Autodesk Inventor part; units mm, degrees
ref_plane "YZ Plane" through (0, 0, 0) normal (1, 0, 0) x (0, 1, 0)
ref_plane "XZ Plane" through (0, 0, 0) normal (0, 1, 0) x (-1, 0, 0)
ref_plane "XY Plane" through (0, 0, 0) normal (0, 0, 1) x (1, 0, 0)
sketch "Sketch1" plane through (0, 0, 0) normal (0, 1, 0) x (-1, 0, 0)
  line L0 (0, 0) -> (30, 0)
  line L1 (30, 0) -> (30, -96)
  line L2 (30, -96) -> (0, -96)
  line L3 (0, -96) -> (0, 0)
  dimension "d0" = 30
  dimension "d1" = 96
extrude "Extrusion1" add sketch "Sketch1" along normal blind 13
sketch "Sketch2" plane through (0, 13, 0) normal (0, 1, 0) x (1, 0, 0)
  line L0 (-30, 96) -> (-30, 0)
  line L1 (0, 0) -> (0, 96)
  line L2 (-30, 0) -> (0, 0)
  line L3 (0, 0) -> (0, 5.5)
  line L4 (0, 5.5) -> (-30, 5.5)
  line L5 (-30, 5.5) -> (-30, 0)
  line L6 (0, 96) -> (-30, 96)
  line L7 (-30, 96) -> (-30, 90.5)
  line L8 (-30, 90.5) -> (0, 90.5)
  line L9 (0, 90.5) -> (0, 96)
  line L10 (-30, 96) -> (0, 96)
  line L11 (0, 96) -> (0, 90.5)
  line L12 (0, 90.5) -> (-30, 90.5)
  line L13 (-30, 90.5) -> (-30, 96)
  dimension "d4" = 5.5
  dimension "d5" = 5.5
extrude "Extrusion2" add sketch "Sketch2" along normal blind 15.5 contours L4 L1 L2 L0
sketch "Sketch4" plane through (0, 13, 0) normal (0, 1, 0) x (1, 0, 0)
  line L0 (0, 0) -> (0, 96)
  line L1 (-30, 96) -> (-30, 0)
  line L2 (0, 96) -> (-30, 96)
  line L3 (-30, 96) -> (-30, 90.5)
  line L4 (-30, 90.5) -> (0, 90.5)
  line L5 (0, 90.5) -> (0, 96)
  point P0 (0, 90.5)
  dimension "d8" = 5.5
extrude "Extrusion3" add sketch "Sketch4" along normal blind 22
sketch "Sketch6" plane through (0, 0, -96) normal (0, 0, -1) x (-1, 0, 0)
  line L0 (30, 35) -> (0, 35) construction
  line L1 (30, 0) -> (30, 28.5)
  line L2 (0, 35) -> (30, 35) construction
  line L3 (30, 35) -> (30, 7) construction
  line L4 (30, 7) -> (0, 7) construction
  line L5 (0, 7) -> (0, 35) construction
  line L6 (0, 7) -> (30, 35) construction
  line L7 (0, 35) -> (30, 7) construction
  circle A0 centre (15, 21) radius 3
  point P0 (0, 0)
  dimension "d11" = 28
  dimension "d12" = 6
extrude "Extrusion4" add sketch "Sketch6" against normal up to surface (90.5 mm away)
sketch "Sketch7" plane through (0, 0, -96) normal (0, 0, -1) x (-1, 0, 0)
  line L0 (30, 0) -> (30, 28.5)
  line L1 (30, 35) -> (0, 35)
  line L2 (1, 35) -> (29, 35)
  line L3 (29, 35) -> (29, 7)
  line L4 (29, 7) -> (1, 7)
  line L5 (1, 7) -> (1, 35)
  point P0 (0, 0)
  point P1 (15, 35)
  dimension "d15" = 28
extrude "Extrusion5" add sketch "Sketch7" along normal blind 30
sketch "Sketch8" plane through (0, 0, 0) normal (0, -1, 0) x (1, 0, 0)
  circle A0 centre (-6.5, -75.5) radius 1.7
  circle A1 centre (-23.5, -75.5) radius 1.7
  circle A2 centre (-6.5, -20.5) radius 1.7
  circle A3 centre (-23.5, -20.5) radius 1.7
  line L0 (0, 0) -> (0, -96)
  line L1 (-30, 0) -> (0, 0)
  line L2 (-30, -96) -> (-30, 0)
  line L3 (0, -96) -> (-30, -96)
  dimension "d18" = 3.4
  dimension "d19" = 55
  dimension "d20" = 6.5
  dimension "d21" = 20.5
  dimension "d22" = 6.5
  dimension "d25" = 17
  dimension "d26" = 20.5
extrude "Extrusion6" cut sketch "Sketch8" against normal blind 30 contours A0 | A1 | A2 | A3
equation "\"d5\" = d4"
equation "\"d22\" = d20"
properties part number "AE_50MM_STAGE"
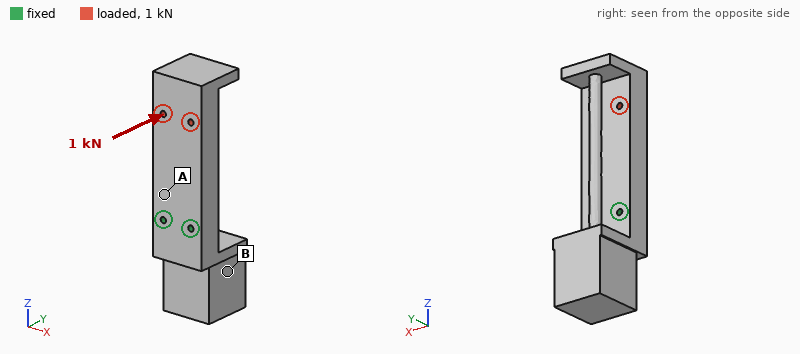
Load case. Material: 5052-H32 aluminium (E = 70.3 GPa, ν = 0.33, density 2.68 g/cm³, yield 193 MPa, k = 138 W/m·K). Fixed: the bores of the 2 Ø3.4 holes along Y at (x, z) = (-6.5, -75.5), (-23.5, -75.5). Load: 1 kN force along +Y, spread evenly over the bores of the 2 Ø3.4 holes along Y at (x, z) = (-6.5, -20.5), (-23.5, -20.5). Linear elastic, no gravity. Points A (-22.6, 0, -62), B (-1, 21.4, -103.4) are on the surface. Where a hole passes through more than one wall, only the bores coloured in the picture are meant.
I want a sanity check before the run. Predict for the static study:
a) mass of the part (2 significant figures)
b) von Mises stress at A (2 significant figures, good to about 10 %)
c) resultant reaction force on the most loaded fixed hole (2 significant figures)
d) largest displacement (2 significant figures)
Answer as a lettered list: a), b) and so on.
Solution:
a) 190 g
b) 42 MPa
c) 510 N
d) 0.20 mm
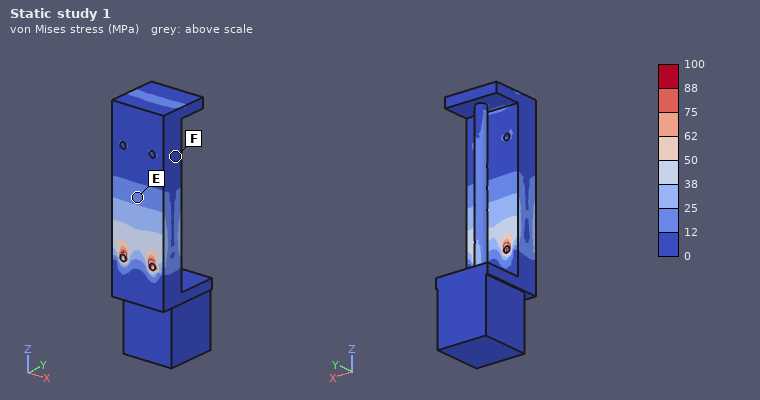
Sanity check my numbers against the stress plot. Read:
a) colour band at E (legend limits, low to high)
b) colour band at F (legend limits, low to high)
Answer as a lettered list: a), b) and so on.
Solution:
a) 12 to 25 MPa
b) 0 to 12 MPa
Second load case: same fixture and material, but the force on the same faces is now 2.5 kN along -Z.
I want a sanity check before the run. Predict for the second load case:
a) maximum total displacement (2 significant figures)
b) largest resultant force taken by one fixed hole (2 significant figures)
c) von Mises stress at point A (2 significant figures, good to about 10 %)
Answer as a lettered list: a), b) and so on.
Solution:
a) 7.4 µm
b) 1.3 kN
c) 7.2 MPa
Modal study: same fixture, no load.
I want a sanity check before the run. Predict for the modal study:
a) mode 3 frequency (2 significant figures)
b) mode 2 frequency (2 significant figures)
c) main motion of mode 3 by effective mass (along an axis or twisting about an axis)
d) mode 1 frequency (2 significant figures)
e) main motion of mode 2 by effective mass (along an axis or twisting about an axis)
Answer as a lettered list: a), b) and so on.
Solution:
a) 3000 Hz
b) 2500 Hz
c) along X
d) 1600 Hz
e) along Y
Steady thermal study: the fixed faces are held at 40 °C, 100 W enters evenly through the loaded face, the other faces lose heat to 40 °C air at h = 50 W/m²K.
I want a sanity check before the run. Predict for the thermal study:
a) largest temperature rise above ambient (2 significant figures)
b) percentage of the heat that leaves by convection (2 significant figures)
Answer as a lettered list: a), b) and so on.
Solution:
a) 84 K
b) 25 %
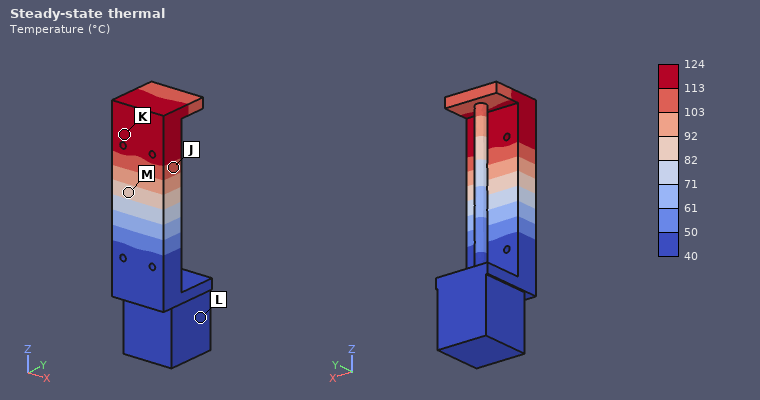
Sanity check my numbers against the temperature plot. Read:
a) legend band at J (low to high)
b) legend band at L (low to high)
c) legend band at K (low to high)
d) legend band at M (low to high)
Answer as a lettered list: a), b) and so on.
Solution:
a) 103 to 113 °C
b) 40 to 50 °C
c) 113 to 124 °C
d) 82 to 92 °C
